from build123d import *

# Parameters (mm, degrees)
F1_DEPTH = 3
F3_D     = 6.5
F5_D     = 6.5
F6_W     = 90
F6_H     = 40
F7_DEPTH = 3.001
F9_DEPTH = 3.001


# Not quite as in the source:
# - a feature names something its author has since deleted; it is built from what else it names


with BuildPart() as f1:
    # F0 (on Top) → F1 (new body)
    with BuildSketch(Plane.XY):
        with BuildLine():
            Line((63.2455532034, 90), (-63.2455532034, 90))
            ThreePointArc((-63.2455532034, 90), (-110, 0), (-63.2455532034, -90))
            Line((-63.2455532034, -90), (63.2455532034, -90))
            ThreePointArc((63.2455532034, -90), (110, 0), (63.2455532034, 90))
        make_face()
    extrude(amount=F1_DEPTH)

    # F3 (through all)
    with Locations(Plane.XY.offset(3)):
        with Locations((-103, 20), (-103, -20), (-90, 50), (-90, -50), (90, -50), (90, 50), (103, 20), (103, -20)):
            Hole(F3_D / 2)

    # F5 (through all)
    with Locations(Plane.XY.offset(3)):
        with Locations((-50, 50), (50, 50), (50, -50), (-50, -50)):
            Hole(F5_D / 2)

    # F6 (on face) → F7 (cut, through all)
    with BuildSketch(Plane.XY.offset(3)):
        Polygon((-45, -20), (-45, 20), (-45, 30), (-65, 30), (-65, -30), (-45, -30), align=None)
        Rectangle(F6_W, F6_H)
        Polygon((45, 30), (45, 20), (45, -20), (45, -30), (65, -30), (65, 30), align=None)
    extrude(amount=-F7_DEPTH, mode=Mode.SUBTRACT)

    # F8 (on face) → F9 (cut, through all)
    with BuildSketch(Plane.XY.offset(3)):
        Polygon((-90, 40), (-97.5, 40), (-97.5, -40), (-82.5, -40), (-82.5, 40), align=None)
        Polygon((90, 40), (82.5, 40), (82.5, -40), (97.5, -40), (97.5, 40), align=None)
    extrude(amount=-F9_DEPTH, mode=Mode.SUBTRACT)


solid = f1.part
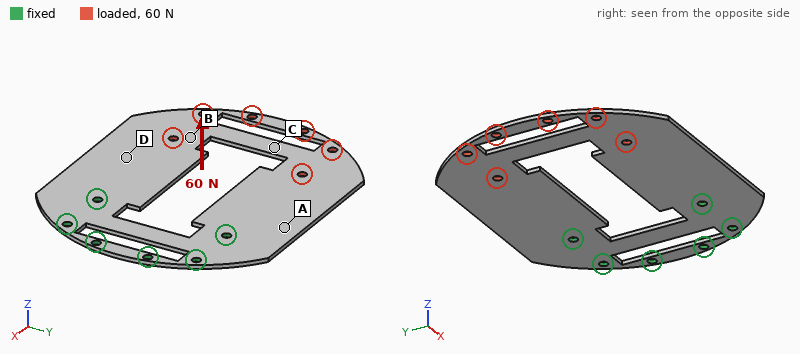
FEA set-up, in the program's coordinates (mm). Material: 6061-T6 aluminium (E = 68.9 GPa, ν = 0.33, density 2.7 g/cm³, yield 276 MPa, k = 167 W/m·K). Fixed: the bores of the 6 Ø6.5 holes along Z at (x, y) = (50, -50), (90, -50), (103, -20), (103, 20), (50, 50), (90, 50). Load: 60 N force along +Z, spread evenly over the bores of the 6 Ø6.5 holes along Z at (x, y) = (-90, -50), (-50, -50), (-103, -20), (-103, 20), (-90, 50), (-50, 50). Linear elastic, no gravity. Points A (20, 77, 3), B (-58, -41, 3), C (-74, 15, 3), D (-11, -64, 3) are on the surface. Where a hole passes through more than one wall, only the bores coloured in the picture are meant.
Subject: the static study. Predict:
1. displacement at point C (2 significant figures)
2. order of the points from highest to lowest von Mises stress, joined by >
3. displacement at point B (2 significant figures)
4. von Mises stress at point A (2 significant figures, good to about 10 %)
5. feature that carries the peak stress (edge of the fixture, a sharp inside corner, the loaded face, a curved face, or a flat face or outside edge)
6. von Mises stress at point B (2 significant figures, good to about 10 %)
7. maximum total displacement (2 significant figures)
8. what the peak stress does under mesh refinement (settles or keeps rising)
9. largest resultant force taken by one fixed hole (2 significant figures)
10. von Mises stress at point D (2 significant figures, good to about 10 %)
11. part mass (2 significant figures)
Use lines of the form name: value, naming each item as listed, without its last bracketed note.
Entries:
displacement at point C: 2.1 mm
order of the points from highest to lowest von Mises stress, joined by >: A > D > B > C
displacement at point B: 1.7 mm
von Mises stress at point A: 28 MPa
feature that carries the peak stress: edge of the fixture
von Mises stress at point B: 12 MPa
maximum total displacement: 3.1 mm
what the peak stress does under mesh refinement: keeps rising
largest resultant force taken by one fixed hole: 59 N
von Mises stress at point D: 20 MPa
part mass: 210 g
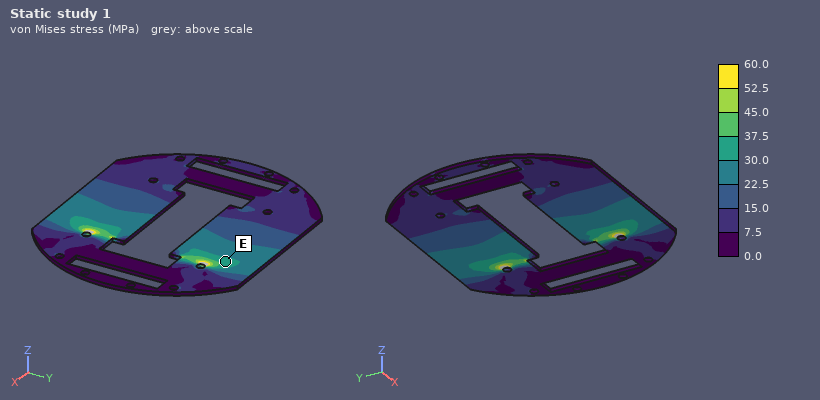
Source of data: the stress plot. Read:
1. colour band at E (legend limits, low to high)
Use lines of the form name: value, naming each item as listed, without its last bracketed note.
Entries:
colour band at E: 30.0 to 37.5 MPa
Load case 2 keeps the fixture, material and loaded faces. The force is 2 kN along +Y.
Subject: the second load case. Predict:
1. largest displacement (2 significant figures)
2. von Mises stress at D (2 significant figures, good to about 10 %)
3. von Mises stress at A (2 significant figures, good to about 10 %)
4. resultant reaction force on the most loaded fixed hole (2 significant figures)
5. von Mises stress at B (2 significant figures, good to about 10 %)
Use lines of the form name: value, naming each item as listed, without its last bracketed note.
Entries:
largest displacement: 0.37 mm
von Mises stress at D: 14 MPa
von Mises stress at A: 25 MPa
resultant reaction force on the most loaded fixed hole: 3.2 kN
von Mises stress at B: 18 MPa
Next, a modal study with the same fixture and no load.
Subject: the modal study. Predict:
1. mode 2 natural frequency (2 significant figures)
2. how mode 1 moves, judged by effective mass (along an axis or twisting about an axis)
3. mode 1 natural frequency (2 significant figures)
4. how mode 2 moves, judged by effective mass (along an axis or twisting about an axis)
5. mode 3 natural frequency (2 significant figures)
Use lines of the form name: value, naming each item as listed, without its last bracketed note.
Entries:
mode 2 natural frequency: 220 Hz
how mode 1 moves, judged by effective mass: along Z
mode 1 natural frequency: 110 Hz
how mode 2 moves, judged by effective mass: twisting about X
mode 3 natural frequency: 520 Hz
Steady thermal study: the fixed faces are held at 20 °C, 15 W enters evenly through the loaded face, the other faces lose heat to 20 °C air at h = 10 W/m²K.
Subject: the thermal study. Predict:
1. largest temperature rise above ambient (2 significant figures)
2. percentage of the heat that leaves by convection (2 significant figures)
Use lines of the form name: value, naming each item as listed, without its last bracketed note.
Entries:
largest temperature rise above ambient: 47 K
percentage of the heat that leaves by convection: 39 %
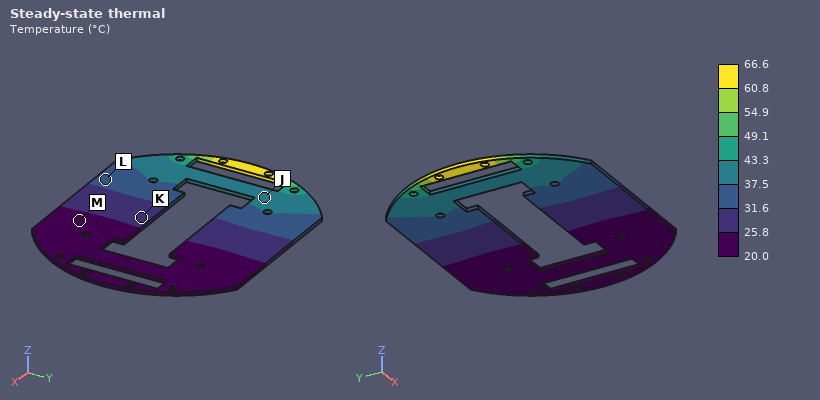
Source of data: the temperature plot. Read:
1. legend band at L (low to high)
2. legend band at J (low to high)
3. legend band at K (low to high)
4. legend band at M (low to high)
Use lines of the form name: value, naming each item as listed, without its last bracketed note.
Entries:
legend band at L: 31.6 to 37.5 °C
legend band at J: 37.5 to 43.3 °C
legend band at K: 25.8 to 31.6 °C
legend band at M: 20.0 to 25.8 °C
